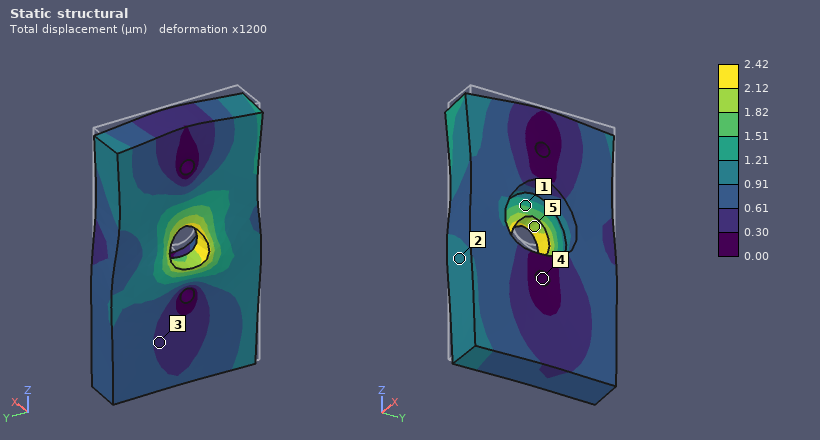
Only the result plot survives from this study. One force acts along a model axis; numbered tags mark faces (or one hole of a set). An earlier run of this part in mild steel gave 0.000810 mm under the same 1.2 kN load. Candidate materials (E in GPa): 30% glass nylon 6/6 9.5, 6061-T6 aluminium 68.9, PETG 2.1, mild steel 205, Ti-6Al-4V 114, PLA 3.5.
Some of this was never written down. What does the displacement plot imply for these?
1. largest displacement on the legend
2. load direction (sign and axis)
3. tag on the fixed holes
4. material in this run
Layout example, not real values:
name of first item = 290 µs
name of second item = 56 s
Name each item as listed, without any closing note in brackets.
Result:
largest displacement on the legend = 2.42 µm
load direction = -Z
tag on the fixed holes = 4
material in this run = 6061-T6 aluminium
